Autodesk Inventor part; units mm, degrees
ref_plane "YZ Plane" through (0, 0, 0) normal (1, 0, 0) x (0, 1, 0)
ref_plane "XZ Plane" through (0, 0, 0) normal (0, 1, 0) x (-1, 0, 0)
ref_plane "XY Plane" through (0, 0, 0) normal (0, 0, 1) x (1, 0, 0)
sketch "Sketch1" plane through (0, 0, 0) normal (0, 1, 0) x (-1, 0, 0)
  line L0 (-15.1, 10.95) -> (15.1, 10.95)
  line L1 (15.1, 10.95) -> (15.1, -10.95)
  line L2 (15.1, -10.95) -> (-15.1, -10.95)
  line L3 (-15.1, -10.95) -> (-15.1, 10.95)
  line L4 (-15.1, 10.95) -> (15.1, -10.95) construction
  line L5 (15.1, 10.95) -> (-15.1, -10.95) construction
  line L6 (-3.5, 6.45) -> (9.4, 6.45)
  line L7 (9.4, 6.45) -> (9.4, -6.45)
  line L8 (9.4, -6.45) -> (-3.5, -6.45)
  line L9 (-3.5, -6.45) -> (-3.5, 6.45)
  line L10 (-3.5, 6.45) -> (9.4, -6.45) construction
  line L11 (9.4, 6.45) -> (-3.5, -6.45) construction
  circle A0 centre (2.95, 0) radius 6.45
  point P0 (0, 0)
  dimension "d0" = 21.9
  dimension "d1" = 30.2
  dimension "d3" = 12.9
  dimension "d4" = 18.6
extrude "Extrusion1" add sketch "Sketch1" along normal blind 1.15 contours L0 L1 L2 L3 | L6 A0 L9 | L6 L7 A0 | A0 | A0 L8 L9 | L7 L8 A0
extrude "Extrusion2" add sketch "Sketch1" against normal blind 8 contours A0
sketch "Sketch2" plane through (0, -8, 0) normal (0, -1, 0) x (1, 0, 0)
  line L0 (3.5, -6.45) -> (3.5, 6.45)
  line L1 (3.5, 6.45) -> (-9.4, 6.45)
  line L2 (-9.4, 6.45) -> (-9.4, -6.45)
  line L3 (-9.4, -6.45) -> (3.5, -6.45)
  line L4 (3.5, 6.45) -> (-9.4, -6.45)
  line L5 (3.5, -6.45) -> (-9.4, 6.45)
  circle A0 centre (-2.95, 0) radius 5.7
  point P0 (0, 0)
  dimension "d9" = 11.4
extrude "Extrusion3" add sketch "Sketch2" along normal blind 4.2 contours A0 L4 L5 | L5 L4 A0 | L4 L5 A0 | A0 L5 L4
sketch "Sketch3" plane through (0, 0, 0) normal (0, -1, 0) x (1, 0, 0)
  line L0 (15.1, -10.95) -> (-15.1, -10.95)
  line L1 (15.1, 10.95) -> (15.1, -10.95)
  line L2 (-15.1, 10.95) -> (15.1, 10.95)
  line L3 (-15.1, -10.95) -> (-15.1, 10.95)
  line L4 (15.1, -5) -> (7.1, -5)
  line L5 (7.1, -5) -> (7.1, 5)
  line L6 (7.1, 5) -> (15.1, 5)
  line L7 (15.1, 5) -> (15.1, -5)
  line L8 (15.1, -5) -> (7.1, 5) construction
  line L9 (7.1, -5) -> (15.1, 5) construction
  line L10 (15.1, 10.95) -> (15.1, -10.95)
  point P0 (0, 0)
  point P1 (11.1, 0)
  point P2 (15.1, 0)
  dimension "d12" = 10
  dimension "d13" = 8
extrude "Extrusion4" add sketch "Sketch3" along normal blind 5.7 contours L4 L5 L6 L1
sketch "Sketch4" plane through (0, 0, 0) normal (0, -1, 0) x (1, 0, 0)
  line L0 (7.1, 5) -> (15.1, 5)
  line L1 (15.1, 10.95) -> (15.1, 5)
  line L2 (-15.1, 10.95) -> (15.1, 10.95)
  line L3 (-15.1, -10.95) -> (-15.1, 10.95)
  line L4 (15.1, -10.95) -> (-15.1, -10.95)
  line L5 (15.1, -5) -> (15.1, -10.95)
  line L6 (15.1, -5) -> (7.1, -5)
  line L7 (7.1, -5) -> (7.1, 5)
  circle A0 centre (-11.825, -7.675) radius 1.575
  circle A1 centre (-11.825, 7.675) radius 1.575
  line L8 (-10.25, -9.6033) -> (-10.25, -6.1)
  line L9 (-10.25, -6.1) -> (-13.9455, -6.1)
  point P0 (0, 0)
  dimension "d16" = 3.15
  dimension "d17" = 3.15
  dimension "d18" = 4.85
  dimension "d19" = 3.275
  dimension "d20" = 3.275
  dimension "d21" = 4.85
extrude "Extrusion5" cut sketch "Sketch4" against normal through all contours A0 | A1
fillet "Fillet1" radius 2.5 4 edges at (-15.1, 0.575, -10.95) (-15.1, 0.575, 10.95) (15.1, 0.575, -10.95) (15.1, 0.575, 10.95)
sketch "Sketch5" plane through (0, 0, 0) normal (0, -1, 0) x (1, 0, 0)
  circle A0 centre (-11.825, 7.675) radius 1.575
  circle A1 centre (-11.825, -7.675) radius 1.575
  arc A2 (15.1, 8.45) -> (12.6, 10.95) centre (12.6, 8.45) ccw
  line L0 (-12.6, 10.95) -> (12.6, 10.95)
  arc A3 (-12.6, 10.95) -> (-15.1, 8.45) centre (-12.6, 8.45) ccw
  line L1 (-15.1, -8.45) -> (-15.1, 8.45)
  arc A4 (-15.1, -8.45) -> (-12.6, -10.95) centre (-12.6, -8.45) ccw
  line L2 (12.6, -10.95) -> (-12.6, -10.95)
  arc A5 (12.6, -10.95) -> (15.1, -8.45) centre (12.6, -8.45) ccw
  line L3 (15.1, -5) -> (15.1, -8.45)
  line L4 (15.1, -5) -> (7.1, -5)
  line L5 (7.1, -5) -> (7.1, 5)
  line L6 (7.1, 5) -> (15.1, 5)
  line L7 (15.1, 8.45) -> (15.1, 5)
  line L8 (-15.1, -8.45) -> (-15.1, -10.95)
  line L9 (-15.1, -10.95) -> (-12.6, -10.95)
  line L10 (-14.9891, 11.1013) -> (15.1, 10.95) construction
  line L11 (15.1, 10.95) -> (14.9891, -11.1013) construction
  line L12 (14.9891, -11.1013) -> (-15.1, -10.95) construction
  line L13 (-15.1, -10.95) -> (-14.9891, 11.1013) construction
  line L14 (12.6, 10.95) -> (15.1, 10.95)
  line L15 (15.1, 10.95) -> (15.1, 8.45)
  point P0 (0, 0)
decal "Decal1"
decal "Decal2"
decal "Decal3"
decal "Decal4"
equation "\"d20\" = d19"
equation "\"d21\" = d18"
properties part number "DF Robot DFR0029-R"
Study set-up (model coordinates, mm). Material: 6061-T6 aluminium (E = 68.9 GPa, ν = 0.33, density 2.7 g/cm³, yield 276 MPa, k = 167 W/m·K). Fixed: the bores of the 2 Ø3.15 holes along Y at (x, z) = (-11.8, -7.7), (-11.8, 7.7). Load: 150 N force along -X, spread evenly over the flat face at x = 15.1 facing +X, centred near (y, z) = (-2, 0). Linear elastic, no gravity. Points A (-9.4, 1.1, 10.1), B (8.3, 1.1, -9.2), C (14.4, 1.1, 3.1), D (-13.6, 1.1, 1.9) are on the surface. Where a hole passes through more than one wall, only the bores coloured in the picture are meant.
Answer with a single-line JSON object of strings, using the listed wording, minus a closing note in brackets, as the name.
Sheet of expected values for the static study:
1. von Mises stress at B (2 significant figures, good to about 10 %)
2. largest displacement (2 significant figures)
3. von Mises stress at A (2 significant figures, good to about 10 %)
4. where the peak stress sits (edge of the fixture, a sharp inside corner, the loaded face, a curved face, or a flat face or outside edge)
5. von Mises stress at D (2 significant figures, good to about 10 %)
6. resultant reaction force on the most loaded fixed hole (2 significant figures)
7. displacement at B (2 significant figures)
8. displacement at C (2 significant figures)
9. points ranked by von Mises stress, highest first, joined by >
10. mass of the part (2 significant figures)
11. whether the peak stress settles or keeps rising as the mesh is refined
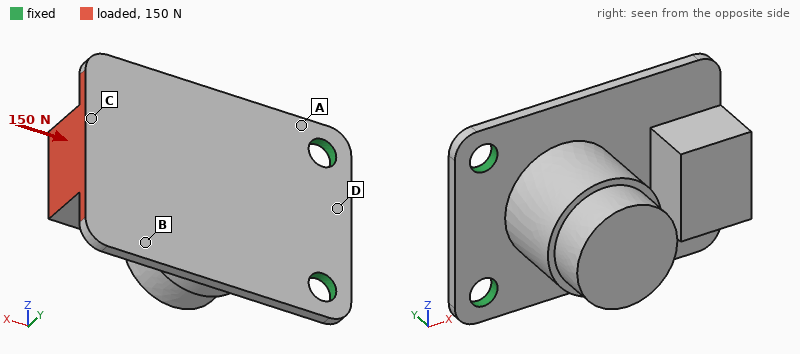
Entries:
{"von Mises stress at B": "36 MPa", "largest displacement": "0.31 mm", "von Mises stress at A": "53 MPa", "where the peak stress sits": "edge of the fixture", "von Mises stress at D": "24 MPa", "resultant reaction force on the most loaded fixed hole": "77 N", "displacement at B": "0.16 mm", "displacement at C": "0.27 mm", "points ranked by von Mises stress, highest first, joined by >": "A > B > D > C", "mass of the part": "7.2 g", "whether the peak stress settles or keeps rising as the mesh is refined": "keeps rising"}
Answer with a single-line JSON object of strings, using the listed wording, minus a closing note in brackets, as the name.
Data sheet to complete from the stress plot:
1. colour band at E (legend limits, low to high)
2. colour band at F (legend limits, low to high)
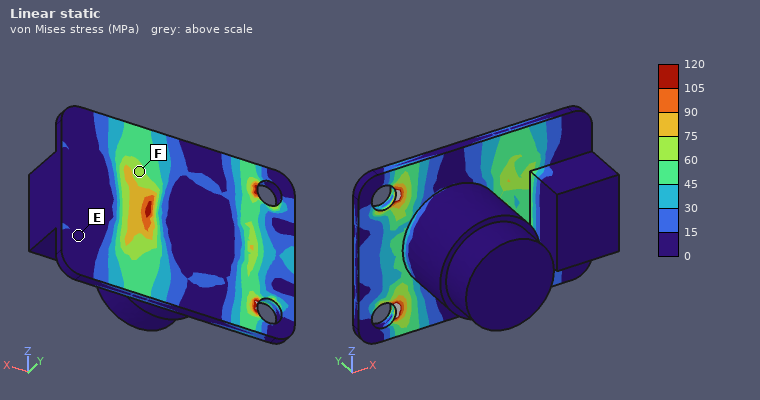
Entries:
{"colour band at E": "0 to 15 MPa", "colour band at F": "60 to 75 MPa"}
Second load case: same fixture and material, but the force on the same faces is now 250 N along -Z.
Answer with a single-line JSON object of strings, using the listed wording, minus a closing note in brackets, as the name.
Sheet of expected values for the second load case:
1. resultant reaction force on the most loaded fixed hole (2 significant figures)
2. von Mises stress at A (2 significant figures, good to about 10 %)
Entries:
{"resultant reaction force on the most loaded fixed hole": "430 N", "von Mises stress at A": "68 MPa"}
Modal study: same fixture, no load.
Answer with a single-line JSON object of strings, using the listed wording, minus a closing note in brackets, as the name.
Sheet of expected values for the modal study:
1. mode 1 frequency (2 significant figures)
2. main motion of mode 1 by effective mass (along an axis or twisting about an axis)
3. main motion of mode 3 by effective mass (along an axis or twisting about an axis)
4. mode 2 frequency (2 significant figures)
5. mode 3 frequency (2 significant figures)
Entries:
{"mode 1 frequency": "1000 Hz", "main motion of mode 1 by effective mass": "along Y", "main motion of mode 3 by effective mass": "along Z", "mode 2 frequency": "4400 Hz", "mode 3 frequency": "5200 Hz"}
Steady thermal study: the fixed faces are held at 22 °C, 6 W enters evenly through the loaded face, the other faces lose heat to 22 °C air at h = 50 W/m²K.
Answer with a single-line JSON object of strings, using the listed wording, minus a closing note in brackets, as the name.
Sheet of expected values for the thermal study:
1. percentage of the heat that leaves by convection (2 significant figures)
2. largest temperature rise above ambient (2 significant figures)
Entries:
{"percentage of the heat that leaves by convection": "19 %", "largest temperature rise above ambient": "24 K"}
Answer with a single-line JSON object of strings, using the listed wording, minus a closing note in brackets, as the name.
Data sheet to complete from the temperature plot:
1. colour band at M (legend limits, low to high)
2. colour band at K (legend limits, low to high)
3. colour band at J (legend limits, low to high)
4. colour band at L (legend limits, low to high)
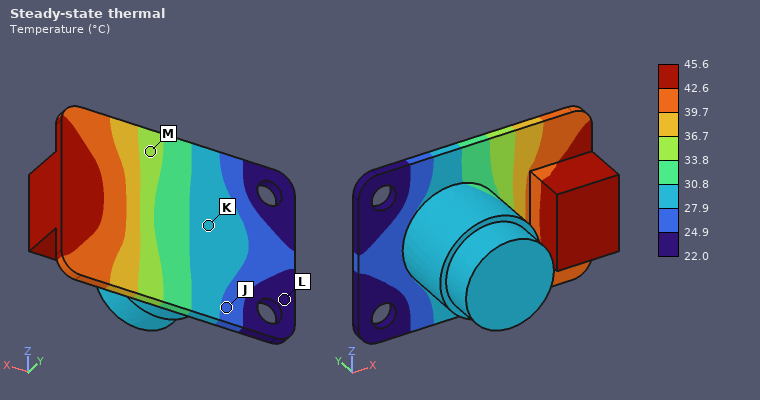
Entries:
{"colour band at M": "33.8 to 36.7 °C", "colour band at K": "27.9 to 30.8 °C", "colour band at J": "24.9 to 27.9 °C", "colour band at L": "22.0 to 24.9 °C"}
